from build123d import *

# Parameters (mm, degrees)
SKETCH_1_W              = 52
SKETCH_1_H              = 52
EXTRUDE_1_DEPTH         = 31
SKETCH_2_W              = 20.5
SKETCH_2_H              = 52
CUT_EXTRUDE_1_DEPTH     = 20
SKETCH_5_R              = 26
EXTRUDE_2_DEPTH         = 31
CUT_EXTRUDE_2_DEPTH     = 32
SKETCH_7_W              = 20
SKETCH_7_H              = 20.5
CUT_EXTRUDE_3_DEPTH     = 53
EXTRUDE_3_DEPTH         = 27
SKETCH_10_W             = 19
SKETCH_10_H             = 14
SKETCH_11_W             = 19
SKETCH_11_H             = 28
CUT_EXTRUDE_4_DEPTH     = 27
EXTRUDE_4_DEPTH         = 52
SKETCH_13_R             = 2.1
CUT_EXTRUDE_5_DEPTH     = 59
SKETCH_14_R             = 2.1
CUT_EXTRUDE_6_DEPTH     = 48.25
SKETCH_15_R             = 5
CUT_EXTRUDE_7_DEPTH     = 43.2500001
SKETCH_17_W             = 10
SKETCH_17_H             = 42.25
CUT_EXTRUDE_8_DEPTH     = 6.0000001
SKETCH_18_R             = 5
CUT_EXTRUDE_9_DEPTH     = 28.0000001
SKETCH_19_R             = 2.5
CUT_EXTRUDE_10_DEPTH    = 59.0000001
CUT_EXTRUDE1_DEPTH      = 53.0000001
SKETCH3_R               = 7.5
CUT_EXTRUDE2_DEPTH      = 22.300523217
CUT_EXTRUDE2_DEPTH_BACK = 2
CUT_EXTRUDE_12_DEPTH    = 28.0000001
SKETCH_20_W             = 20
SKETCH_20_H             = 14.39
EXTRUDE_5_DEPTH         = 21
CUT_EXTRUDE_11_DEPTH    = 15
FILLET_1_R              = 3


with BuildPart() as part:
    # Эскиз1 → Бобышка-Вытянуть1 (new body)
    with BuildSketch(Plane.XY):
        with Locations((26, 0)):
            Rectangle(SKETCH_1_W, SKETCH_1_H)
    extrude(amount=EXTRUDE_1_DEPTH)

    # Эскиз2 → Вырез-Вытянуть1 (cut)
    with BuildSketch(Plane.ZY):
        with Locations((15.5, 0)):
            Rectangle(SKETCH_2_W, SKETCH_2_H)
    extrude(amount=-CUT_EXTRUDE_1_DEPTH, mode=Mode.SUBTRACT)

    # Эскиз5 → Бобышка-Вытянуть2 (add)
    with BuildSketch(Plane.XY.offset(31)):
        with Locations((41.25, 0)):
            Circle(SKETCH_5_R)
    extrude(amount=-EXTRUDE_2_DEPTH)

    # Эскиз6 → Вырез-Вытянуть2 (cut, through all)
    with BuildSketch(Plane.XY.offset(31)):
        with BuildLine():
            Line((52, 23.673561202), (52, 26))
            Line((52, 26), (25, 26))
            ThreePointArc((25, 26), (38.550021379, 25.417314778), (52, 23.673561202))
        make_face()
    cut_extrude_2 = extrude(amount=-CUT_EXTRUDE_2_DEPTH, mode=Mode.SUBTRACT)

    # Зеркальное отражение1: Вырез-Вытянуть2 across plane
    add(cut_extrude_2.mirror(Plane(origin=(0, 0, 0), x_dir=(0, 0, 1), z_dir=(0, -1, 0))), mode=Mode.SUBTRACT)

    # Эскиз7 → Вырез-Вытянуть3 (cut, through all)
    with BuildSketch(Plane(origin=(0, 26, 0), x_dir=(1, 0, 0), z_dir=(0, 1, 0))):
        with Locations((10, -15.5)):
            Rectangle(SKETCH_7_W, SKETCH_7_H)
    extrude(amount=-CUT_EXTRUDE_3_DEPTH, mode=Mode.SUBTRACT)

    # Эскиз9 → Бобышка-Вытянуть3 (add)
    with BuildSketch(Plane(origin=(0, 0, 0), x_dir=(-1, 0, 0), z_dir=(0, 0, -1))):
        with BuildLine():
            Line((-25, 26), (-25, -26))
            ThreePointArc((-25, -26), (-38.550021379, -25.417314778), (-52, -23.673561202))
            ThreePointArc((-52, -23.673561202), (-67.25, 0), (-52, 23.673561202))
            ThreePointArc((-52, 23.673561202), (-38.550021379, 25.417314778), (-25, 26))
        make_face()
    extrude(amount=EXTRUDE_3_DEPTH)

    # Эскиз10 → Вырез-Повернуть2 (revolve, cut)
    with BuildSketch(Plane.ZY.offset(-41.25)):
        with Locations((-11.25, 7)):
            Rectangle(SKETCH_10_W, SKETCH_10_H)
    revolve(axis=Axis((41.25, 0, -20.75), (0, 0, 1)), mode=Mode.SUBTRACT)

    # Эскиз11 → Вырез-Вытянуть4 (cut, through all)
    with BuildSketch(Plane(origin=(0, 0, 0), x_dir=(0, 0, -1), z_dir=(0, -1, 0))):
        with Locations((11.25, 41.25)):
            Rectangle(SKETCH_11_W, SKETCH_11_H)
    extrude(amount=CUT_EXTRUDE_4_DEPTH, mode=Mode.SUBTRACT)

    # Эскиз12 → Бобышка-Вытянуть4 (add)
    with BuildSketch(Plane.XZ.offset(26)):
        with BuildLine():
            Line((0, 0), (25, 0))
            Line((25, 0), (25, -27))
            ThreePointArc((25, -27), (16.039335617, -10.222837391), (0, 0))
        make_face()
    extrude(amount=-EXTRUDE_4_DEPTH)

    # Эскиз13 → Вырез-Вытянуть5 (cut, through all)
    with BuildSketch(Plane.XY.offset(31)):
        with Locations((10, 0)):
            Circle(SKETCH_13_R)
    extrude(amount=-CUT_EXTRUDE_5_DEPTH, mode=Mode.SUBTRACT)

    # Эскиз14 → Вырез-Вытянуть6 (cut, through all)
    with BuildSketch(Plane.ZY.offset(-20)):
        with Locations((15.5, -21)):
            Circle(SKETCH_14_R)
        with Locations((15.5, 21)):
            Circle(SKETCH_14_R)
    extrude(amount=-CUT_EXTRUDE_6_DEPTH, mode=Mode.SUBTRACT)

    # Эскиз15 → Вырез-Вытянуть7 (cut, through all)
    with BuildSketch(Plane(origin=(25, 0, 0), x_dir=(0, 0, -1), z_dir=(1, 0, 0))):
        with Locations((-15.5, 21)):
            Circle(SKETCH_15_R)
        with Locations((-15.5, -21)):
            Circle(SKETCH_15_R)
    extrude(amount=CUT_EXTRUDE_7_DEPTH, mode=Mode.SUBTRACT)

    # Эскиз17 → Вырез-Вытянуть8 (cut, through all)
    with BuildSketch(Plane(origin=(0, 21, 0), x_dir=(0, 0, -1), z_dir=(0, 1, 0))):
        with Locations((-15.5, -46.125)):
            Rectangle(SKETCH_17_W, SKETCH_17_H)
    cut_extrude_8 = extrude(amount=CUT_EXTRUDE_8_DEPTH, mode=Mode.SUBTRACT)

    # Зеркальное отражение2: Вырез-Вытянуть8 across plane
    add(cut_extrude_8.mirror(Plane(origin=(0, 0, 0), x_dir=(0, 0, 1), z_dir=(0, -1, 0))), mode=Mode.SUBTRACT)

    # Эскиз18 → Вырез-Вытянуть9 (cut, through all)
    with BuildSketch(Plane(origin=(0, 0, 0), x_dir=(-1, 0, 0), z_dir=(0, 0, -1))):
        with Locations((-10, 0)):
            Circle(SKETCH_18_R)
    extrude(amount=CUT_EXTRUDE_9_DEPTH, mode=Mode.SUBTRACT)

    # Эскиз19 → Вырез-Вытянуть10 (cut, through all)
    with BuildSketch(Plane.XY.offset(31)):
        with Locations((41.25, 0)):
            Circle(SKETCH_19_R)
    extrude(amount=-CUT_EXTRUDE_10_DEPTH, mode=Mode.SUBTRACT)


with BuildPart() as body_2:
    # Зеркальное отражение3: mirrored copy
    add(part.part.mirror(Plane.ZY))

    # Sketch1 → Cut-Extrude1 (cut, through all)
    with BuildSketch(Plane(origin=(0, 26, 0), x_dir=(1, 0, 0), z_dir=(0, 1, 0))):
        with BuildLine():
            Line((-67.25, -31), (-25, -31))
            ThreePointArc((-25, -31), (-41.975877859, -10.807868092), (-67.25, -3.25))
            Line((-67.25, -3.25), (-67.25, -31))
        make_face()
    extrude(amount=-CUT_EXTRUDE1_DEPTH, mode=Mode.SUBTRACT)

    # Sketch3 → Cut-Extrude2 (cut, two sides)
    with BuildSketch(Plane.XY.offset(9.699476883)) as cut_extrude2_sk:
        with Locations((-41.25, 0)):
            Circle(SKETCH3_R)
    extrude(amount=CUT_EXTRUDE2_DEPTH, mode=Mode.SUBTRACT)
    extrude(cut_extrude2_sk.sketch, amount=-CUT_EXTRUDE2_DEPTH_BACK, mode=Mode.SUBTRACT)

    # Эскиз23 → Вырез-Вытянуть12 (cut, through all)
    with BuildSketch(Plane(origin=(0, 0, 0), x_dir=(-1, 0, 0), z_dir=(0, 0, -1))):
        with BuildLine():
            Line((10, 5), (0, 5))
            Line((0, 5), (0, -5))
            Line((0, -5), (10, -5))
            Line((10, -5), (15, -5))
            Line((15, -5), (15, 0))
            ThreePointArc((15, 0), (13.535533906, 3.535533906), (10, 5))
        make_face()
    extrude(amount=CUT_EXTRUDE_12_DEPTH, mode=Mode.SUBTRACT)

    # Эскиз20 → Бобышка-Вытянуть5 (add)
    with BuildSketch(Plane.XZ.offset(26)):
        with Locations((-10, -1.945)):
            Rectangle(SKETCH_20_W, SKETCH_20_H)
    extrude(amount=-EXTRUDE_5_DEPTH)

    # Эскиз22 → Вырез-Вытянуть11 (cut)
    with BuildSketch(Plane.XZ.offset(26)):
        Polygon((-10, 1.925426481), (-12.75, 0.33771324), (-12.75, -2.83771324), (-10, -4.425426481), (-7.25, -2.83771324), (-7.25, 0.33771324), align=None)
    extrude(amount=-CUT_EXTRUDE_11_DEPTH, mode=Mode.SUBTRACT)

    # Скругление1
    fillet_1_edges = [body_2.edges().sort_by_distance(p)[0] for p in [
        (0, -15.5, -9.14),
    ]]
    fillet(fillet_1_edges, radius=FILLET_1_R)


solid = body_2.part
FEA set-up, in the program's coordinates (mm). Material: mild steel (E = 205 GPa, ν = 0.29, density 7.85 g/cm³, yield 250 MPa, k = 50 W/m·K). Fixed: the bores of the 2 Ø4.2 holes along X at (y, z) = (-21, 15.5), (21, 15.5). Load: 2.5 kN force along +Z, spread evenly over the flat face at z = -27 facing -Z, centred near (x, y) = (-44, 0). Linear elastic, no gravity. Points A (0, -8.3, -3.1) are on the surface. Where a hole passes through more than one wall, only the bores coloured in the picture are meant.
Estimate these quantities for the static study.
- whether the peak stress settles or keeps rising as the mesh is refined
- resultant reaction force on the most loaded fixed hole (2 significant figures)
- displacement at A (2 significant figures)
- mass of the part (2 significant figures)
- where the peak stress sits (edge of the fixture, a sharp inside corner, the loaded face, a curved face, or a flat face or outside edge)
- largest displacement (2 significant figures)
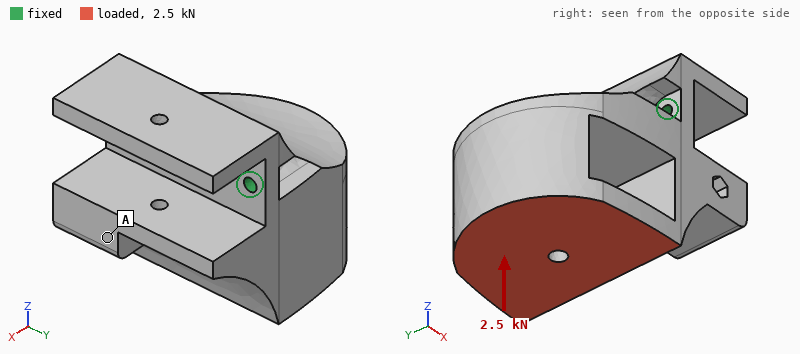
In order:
keeps rising
1.3 kN
0.052 mm
650 g
edge of the fixture
0.11 mm
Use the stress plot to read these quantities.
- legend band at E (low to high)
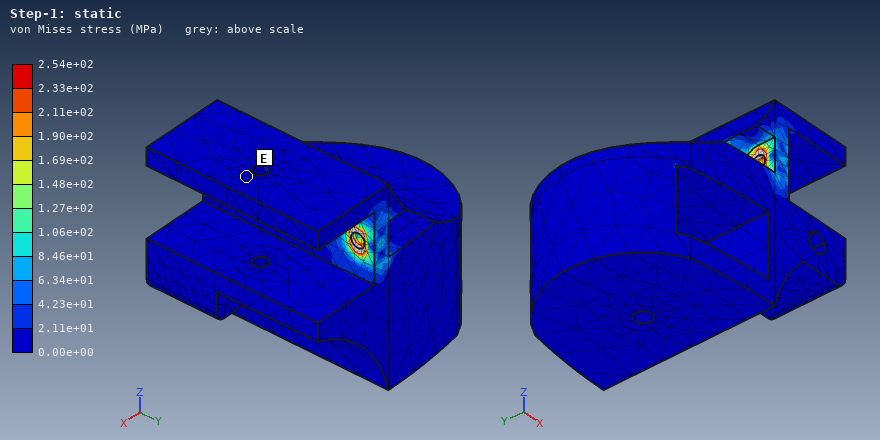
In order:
0.00e+00 to 2.11e+01 MPa
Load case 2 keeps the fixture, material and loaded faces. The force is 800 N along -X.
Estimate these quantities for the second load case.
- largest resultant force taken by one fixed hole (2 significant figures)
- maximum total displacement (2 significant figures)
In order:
420 N
72 µm
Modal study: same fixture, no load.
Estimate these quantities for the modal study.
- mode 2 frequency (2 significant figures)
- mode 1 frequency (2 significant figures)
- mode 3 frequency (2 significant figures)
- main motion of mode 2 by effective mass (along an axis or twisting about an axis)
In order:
5100 Hz
1100 Hz
6400 Hz
along Y
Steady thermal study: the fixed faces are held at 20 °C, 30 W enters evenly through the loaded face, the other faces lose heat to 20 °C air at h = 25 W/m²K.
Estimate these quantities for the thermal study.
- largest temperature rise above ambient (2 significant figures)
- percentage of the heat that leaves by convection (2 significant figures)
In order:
41 K
32 %
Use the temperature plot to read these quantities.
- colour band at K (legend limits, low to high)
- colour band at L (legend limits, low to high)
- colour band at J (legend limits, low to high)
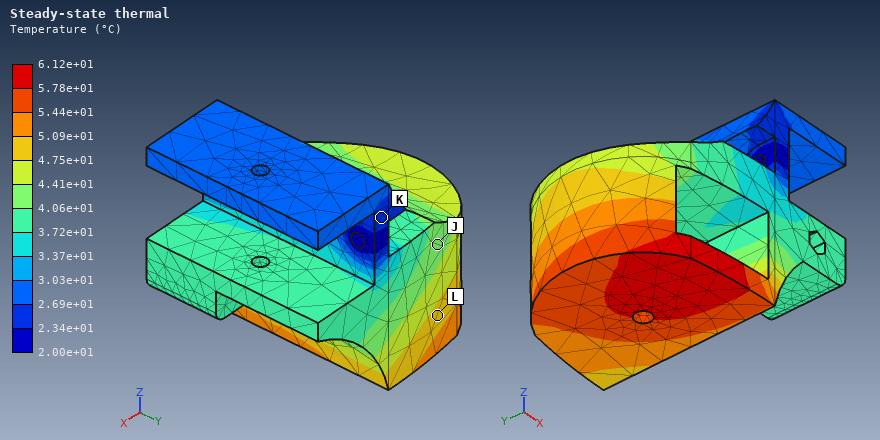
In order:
2.34e+01 to 2.69e+01 °C
4.75e+01 to 5.09e+01 °C
4.06e+01 to 4.41e+01 °C
